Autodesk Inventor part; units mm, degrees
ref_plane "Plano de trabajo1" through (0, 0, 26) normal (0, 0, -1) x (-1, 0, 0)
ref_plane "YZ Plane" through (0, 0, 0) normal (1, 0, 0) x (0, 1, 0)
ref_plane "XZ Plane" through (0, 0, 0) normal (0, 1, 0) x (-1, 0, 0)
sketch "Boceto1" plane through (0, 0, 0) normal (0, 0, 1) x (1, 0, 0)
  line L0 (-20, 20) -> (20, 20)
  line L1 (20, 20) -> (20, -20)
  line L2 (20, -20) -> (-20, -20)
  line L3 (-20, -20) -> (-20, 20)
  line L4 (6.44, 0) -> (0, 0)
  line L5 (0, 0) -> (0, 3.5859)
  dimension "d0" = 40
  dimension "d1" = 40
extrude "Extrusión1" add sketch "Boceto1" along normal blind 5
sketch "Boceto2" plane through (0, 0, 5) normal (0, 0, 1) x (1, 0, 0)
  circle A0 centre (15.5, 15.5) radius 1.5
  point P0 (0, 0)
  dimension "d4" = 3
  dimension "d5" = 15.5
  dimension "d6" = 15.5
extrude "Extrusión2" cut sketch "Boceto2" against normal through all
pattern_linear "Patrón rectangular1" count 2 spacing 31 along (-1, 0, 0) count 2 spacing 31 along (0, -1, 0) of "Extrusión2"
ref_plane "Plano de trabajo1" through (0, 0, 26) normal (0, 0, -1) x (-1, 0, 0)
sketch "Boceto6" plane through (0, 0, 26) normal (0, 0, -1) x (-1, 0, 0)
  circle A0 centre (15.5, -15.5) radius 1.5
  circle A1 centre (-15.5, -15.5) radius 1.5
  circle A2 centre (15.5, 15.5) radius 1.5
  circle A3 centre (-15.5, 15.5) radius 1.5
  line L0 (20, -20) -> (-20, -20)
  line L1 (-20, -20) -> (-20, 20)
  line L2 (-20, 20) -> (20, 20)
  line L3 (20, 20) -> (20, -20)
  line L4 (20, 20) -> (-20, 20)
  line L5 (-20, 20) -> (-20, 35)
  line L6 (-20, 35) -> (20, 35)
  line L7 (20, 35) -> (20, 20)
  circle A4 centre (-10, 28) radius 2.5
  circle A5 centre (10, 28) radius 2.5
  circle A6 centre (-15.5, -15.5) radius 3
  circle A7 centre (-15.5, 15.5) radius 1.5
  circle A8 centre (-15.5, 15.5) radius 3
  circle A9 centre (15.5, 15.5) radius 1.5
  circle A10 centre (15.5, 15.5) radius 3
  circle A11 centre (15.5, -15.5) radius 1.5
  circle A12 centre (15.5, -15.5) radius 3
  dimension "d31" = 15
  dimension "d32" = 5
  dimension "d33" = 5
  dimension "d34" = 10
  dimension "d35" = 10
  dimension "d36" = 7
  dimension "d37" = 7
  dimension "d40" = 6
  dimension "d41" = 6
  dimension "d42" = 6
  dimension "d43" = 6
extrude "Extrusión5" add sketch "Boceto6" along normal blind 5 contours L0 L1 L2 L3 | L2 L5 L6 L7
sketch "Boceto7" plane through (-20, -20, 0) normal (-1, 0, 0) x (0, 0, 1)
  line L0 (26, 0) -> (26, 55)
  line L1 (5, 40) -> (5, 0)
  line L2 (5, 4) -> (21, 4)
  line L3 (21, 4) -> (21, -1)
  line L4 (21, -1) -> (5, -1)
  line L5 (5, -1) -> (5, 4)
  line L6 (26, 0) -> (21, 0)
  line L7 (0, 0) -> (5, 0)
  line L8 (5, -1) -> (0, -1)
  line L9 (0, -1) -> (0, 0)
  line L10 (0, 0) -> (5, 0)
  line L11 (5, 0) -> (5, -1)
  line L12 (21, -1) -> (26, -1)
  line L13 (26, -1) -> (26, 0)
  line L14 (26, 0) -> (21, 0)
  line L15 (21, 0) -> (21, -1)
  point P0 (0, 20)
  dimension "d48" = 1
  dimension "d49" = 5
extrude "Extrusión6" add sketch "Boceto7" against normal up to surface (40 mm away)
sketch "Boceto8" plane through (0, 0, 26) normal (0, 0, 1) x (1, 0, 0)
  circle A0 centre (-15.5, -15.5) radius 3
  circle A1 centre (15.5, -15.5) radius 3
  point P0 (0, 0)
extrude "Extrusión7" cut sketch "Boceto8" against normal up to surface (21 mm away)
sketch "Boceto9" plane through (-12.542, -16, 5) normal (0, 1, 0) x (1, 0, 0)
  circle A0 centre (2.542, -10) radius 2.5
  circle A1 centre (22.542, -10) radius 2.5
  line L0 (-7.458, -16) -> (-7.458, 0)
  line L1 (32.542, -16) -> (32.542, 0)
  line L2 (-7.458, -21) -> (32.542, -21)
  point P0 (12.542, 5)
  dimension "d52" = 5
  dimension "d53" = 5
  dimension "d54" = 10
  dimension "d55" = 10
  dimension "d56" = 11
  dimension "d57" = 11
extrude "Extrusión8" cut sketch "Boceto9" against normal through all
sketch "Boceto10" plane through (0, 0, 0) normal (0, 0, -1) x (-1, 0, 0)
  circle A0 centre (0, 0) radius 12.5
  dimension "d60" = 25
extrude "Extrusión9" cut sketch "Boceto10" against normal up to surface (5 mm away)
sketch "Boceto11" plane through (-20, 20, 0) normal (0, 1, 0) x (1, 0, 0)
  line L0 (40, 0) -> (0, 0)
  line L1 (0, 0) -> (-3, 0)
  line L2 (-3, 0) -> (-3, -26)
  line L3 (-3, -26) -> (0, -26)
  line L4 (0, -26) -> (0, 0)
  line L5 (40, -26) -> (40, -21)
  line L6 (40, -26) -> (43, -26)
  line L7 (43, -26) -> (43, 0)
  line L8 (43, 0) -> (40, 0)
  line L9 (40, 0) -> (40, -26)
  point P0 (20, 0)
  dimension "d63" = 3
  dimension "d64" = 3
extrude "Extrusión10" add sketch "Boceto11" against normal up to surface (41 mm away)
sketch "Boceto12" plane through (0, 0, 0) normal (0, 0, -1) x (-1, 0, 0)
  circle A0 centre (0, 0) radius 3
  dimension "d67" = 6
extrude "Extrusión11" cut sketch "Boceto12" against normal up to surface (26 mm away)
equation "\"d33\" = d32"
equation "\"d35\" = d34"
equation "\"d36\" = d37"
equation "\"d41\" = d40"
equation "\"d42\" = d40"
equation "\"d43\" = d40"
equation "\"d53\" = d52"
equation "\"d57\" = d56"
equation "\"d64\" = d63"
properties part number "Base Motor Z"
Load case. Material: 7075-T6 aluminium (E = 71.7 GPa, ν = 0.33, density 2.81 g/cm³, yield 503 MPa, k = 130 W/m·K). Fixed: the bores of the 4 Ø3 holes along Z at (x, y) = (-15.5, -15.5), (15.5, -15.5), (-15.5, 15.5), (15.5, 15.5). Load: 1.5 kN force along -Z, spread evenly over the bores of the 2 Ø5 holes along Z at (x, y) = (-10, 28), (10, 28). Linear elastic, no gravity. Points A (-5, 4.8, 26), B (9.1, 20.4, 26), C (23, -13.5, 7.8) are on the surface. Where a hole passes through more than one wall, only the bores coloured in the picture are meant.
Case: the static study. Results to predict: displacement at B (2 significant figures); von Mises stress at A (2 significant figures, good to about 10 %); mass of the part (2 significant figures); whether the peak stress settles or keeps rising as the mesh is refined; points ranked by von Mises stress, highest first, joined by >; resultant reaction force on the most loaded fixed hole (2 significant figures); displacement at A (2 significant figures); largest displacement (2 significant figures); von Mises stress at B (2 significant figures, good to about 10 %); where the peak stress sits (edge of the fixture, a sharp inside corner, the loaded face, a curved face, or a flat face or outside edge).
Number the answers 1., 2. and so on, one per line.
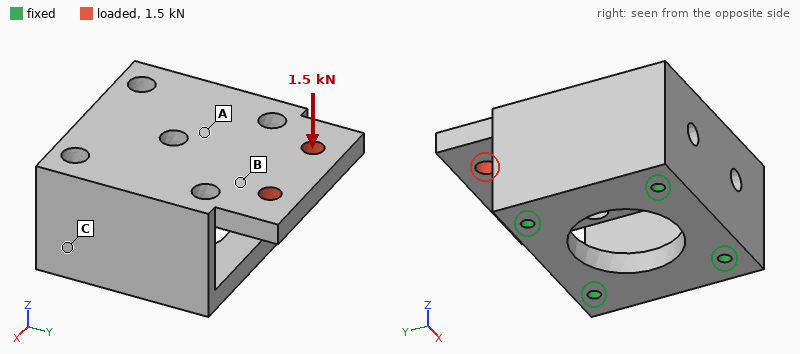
1. 0.12 mm
2. 53 MPa
3. 70 g
4. keeps rising
5. B > A > C
6. 1.0 kN
7. 0.043 mm
8. 0.29 mm
9. 100 MPa
10. a sharp inside corner
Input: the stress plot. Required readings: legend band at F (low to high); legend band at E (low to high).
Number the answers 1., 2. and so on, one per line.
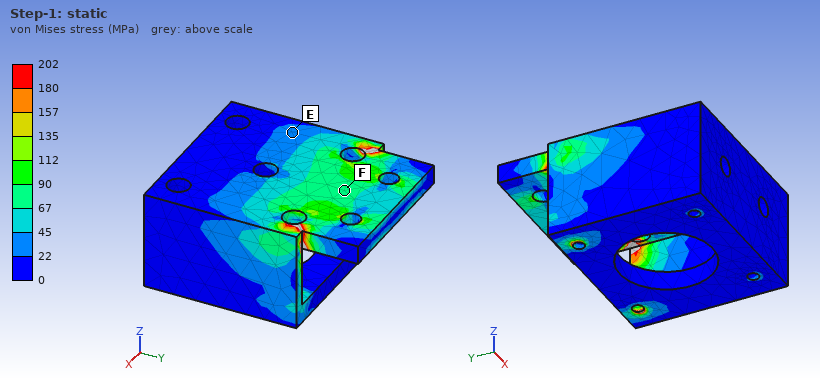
1. 67 to 90 MPa
2. 22 to 45 MPa
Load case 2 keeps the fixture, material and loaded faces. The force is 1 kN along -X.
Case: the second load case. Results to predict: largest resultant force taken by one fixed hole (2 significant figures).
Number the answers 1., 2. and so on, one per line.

1. 1.1 kN
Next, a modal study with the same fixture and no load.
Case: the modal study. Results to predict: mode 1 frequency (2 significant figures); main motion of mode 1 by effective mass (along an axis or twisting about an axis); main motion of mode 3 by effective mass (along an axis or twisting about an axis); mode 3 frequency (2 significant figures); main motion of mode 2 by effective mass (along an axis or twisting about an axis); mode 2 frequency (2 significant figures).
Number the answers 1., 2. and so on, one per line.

1. 4700 Hz
2. along Z
3. along Y
4. 9300 Hz
5. along X
6. 5500 Hz
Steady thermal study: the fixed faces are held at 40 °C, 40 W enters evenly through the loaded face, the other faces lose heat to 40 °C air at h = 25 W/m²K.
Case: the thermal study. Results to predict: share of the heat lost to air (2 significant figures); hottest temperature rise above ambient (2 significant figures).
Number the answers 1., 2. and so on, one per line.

1. 14 %
2. 61 K
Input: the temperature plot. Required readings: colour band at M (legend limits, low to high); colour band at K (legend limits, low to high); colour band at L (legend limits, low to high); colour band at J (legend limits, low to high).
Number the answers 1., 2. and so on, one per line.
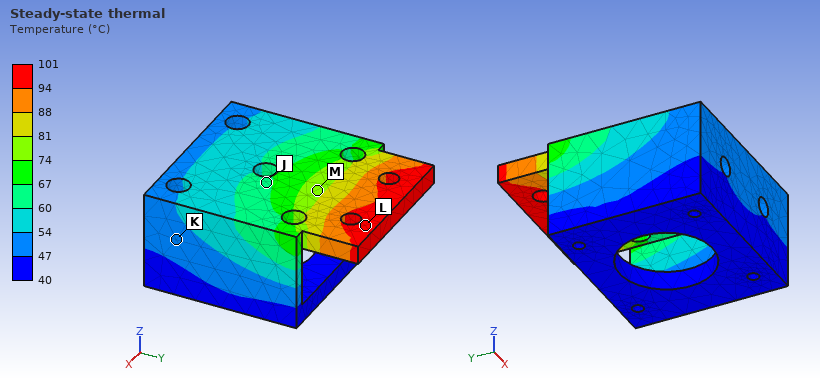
1. 74 to 81 °C
2. 47 to 54 °C
3. 94 to 101 °C
4. 60 to 67 °C
